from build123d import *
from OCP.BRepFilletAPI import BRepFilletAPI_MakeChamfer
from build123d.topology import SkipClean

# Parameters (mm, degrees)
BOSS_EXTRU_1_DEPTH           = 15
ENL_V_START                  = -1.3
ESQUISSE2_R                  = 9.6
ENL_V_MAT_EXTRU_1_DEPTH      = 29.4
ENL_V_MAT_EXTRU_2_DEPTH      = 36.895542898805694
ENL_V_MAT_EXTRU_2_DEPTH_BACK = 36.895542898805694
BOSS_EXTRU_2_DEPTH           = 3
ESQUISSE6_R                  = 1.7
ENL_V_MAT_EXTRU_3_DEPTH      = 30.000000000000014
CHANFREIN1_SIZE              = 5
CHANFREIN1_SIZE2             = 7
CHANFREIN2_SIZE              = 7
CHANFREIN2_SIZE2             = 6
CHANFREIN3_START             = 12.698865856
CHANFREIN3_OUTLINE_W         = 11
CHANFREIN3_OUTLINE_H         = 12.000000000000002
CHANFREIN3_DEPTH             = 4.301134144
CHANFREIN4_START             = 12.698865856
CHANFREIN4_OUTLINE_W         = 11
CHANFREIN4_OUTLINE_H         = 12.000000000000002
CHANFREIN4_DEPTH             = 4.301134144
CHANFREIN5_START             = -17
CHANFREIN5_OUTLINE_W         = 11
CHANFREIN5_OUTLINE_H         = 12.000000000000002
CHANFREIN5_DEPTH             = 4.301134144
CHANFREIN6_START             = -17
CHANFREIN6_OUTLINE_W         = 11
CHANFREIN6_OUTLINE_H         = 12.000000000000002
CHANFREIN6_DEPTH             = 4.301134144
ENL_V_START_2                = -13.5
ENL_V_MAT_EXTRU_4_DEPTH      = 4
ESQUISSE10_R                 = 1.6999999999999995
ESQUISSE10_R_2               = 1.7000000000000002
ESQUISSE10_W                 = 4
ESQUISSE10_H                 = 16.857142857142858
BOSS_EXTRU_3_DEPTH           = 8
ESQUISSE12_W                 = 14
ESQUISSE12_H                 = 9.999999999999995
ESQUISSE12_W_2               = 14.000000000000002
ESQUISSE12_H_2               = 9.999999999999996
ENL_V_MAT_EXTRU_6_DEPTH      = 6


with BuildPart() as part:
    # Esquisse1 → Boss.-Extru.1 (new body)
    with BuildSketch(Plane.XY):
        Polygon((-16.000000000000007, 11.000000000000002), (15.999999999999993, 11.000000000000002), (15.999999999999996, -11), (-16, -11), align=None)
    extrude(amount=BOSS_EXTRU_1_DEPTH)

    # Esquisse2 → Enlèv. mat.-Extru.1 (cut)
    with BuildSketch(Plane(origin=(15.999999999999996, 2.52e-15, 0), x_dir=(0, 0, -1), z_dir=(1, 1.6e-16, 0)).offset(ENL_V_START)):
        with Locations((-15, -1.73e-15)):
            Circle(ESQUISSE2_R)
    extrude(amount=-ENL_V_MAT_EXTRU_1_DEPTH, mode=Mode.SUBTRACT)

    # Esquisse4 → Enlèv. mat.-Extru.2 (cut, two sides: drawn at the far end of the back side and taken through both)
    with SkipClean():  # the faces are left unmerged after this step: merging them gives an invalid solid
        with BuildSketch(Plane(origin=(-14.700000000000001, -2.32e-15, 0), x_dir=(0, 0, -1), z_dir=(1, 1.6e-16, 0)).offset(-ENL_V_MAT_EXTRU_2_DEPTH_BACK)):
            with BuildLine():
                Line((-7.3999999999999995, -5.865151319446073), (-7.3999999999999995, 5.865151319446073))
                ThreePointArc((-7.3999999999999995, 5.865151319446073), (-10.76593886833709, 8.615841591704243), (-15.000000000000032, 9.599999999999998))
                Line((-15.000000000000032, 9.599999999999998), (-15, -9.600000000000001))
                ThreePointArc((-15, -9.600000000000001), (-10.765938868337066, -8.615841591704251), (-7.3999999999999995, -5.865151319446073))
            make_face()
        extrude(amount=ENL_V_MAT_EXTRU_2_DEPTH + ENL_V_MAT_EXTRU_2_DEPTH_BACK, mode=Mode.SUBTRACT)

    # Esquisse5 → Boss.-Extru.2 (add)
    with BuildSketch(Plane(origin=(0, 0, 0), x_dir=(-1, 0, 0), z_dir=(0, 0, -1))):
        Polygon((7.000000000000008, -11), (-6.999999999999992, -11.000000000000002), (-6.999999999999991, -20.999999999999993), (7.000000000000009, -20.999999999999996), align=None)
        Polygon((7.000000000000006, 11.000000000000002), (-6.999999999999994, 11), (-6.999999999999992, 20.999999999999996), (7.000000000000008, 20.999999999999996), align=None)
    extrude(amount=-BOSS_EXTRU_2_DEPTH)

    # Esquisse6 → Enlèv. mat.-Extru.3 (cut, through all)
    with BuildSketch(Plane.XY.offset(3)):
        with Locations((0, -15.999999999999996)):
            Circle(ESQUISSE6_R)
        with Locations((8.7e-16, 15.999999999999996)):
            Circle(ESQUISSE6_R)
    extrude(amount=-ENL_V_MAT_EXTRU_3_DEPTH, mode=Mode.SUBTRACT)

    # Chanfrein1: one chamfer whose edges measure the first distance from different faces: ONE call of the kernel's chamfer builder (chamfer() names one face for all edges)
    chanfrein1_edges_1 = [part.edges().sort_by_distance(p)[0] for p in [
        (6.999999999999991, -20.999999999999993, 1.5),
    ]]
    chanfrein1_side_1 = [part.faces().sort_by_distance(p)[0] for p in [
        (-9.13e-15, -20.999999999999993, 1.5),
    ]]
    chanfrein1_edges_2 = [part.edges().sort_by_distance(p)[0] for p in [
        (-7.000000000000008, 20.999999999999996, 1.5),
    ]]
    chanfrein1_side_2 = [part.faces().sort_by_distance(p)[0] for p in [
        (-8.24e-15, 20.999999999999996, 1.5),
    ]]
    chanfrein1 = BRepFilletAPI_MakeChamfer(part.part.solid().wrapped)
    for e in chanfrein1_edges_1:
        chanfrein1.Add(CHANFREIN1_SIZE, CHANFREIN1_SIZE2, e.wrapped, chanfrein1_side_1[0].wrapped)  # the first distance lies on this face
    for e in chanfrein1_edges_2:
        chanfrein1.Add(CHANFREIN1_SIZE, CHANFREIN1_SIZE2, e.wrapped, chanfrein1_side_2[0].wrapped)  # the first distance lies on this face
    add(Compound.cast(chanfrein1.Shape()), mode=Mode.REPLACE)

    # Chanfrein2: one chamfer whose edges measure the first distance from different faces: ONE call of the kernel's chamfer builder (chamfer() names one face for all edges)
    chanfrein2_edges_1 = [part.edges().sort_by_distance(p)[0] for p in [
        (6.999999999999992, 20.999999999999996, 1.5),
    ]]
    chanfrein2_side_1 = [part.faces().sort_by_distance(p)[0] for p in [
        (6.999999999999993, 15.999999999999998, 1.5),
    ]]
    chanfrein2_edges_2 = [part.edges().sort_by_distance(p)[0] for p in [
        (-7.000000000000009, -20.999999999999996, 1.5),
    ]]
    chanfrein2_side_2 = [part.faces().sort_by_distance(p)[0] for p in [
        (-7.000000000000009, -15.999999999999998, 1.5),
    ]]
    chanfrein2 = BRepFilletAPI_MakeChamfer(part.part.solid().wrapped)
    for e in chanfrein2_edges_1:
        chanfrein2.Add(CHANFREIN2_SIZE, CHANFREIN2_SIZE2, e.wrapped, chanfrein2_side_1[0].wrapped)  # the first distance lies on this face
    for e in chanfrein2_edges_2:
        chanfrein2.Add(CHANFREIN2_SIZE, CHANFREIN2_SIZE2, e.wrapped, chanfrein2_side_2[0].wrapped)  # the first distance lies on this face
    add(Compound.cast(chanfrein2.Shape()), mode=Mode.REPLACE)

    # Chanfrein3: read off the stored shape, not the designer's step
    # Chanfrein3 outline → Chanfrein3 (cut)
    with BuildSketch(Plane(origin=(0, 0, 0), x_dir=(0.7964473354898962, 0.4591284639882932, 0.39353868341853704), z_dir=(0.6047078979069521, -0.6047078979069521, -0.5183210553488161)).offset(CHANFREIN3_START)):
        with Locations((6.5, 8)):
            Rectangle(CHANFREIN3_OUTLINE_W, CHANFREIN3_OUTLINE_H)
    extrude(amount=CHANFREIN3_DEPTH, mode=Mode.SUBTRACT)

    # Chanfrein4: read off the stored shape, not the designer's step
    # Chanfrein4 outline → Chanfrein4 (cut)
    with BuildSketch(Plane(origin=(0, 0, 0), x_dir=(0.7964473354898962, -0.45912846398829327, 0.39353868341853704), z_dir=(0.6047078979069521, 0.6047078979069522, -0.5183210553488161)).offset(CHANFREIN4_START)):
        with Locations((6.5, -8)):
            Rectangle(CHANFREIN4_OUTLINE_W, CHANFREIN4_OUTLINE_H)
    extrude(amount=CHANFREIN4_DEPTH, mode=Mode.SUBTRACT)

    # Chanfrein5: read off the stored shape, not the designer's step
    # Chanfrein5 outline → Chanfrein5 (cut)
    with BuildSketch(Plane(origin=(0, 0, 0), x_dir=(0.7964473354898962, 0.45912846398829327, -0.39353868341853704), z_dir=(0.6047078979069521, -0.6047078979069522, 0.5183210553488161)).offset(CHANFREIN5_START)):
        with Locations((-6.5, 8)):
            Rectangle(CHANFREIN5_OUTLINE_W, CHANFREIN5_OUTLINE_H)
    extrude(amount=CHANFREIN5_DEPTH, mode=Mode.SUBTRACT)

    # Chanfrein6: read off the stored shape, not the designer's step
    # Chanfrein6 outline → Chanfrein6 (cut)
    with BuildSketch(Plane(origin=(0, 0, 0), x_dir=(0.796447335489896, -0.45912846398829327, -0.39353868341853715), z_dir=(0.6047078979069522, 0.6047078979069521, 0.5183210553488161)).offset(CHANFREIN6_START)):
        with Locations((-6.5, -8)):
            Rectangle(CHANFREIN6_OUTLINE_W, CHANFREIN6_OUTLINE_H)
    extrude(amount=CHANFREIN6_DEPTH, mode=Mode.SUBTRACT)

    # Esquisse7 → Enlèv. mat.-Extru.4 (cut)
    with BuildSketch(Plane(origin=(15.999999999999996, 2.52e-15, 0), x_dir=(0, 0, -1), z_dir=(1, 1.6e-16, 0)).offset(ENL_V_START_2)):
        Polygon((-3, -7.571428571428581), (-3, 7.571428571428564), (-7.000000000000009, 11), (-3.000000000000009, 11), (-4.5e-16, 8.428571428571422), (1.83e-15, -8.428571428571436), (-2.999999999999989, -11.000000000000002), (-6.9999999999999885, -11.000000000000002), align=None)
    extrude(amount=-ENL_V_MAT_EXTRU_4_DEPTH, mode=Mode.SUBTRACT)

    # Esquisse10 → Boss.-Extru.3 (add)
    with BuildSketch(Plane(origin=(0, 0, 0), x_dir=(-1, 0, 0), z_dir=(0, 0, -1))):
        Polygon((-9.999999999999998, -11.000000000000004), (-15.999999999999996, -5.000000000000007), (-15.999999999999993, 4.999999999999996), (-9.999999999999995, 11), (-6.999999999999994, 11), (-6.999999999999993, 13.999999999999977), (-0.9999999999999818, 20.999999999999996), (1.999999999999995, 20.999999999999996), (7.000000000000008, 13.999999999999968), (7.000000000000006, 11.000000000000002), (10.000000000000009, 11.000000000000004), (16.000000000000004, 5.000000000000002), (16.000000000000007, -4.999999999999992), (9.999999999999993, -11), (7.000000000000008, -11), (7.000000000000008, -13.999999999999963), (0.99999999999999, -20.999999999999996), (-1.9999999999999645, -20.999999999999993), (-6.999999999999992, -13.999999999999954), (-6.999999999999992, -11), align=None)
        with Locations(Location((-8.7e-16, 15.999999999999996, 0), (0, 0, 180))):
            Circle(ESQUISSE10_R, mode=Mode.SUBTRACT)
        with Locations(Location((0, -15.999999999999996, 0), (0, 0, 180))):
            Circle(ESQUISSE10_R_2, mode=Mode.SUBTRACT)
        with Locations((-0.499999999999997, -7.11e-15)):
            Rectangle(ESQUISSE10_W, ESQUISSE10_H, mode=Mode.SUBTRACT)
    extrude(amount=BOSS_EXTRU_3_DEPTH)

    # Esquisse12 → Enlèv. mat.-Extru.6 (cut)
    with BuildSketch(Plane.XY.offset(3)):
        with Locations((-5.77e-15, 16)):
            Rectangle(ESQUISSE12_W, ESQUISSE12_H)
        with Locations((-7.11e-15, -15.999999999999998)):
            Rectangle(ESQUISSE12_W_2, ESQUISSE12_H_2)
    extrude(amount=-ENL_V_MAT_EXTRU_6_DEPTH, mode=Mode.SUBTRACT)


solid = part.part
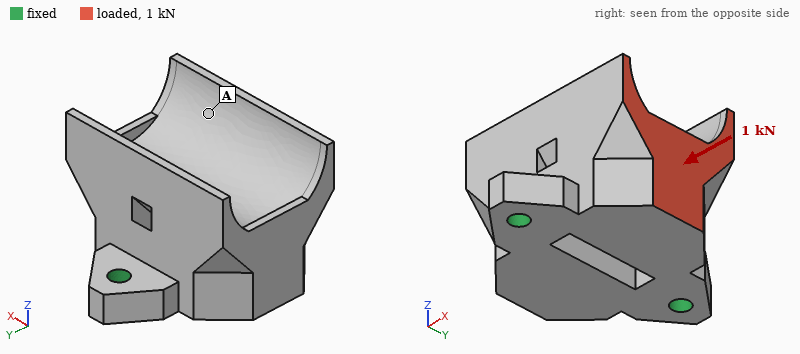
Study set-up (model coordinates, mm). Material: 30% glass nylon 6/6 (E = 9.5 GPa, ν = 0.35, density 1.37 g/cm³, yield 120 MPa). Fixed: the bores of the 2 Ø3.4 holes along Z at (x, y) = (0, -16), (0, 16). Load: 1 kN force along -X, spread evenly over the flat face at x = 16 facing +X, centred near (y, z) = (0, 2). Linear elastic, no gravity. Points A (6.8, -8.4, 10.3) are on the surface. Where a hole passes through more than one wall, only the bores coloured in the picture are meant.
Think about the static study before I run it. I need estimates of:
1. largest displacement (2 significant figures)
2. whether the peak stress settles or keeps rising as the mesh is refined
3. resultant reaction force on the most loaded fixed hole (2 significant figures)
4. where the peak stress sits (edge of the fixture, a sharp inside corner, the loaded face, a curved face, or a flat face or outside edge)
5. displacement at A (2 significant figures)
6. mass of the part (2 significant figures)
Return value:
0.42 mm
keeps rising
500 N
edge of the fixture
0.28 mm
15 g
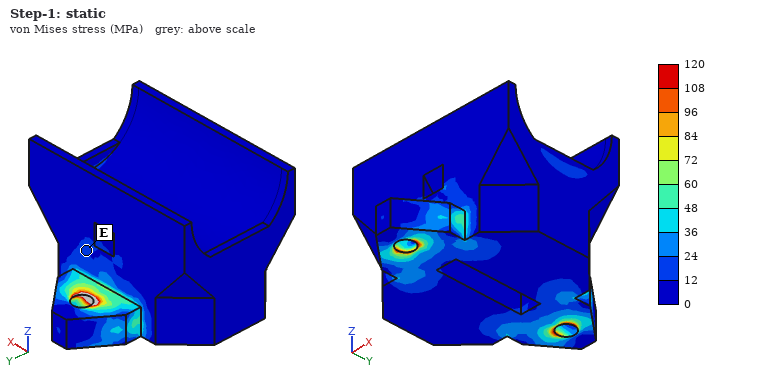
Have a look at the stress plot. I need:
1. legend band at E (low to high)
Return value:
12 to 24 MPa
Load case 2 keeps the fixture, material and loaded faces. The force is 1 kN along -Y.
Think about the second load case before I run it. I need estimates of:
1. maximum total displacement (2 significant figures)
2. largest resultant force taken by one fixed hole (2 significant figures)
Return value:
0.15 mm
780 N
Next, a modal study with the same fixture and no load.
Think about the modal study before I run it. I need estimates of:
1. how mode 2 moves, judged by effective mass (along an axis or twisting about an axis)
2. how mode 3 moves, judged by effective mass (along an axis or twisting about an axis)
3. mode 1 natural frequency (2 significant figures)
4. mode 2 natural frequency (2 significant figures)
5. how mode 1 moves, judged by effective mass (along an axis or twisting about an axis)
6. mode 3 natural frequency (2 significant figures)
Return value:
along Z
along Y
2500 Hz
7200 Hz
along X
8300 Hz
